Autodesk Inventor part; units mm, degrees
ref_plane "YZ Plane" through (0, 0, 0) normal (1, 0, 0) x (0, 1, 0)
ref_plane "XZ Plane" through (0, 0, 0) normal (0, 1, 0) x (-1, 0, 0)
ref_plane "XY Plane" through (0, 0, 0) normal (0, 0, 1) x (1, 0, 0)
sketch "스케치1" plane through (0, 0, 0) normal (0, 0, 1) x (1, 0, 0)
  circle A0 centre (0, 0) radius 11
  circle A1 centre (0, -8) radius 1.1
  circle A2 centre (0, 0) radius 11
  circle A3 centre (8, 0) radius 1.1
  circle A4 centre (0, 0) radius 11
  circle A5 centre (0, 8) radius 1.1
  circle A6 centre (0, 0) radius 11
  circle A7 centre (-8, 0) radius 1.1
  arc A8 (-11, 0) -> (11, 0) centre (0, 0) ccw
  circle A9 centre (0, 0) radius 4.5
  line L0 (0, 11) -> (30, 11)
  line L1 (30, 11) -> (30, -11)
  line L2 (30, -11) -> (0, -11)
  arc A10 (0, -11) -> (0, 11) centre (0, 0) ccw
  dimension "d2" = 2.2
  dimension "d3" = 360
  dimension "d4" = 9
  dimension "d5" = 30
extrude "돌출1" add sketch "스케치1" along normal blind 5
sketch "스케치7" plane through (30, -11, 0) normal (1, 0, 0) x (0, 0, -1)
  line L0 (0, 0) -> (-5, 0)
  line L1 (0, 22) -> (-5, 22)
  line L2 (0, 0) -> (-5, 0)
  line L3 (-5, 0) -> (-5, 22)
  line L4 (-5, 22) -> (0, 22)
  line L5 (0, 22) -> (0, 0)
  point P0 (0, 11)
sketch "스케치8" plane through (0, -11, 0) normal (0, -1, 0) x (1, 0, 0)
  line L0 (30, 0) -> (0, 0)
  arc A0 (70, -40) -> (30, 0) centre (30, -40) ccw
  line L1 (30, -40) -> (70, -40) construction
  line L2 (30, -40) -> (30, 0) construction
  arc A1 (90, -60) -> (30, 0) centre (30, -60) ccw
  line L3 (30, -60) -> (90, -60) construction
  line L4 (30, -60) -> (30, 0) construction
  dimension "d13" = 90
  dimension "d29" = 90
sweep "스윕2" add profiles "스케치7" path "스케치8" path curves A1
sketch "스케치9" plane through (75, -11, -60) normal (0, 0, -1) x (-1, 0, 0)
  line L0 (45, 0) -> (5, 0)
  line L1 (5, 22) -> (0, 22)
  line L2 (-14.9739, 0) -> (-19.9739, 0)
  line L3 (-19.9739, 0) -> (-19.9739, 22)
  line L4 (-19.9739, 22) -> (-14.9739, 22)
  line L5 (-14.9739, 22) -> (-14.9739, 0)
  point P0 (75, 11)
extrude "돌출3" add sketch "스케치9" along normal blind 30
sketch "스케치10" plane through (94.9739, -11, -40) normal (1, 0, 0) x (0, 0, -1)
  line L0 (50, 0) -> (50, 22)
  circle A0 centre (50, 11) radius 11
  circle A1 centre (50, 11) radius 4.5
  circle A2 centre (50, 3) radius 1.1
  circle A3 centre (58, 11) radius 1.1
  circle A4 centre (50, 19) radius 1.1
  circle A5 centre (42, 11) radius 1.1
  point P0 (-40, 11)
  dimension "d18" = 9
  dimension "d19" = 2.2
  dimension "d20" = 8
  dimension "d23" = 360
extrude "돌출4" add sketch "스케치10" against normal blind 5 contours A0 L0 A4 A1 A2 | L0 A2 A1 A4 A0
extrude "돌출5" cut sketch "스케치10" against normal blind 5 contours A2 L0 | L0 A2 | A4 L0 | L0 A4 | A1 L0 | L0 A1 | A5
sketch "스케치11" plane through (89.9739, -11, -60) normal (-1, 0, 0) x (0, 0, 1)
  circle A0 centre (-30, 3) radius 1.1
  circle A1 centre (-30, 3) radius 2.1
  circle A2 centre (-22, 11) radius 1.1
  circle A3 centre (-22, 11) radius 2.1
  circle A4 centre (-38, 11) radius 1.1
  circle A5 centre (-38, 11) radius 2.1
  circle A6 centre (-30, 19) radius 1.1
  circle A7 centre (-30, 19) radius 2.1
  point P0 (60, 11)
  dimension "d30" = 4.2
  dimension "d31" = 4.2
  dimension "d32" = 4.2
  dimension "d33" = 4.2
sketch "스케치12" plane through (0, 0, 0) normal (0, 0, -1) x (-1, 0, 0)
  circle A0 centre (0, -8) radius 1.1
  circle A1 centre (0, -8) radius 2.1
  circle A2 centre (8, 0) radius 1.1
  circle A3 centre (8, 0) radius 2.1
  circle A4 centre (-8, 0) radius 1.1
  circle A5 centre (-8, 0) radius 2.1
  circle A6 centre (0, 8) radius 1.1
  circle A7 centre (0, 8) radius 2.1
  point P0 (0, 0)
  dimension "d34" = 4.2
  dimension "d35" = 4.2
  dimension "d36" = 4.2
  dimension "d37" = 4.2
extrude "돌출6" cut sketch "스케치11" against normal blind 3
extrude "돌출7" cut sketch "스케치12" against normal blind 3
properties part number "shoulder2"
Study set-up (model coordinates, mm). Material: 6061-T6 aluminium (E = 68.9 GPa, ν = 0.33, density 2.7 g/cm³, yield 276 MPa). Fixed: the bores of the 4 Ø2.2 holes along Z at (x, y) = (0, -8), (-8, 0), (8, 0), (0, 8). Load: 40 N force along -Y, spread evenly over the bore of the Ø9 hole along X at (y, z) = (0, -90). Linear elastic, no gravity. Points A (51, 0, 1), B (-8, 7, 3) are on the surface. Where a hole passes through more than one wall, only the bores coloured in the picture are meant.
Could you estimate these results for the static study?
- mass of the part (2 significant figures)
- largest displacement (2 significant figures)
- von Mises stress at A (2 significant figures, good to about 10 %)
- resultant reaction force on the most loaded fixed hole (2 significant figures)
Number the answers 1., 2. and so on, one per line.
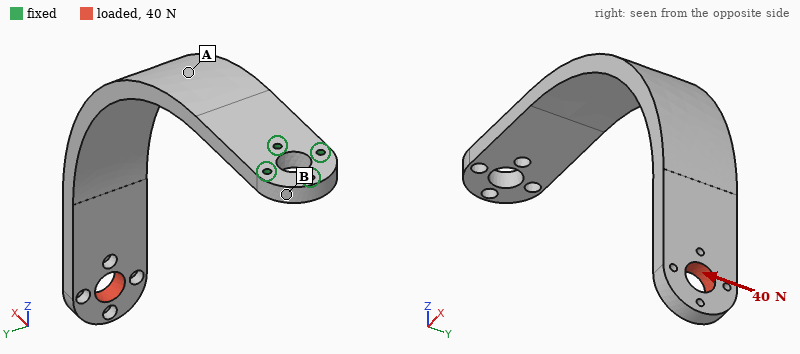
1. 49 g
2. 1.2 mm
3. 28 MPa
4. 320 N
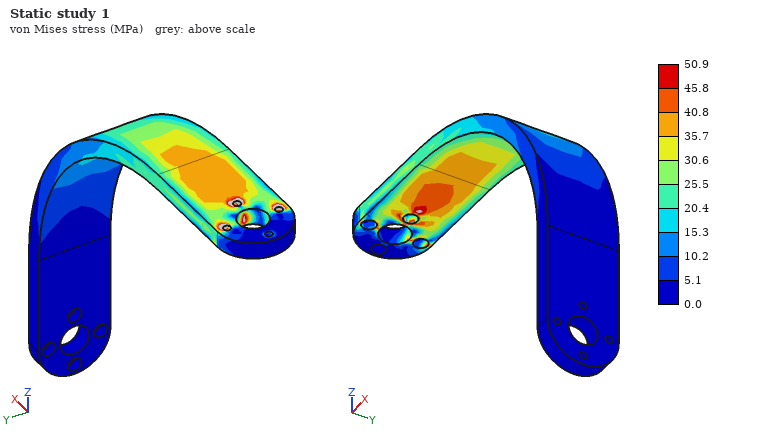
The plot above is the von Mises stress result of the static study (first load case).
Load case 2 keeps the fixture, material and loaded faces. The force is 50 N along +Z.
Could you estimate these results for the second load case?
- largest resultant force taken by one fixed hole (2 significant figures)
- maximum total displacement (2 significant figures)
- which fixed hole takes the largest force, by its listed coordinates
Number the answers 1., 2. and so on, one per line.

1. 560 N
2. 1.5 mm
3. (8, 0)
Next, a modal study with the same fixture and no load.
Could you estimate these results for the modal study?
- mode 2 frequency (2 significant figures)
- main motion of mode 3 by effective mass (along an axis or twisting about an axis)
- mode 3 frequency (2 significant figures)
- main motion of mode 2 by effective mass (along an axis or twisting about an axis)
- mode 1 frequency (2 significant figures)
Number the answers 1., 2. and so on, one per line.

1. 310 Hz
2. along Z
3. 690 Hz
4. along Y
5. 180 Hz
